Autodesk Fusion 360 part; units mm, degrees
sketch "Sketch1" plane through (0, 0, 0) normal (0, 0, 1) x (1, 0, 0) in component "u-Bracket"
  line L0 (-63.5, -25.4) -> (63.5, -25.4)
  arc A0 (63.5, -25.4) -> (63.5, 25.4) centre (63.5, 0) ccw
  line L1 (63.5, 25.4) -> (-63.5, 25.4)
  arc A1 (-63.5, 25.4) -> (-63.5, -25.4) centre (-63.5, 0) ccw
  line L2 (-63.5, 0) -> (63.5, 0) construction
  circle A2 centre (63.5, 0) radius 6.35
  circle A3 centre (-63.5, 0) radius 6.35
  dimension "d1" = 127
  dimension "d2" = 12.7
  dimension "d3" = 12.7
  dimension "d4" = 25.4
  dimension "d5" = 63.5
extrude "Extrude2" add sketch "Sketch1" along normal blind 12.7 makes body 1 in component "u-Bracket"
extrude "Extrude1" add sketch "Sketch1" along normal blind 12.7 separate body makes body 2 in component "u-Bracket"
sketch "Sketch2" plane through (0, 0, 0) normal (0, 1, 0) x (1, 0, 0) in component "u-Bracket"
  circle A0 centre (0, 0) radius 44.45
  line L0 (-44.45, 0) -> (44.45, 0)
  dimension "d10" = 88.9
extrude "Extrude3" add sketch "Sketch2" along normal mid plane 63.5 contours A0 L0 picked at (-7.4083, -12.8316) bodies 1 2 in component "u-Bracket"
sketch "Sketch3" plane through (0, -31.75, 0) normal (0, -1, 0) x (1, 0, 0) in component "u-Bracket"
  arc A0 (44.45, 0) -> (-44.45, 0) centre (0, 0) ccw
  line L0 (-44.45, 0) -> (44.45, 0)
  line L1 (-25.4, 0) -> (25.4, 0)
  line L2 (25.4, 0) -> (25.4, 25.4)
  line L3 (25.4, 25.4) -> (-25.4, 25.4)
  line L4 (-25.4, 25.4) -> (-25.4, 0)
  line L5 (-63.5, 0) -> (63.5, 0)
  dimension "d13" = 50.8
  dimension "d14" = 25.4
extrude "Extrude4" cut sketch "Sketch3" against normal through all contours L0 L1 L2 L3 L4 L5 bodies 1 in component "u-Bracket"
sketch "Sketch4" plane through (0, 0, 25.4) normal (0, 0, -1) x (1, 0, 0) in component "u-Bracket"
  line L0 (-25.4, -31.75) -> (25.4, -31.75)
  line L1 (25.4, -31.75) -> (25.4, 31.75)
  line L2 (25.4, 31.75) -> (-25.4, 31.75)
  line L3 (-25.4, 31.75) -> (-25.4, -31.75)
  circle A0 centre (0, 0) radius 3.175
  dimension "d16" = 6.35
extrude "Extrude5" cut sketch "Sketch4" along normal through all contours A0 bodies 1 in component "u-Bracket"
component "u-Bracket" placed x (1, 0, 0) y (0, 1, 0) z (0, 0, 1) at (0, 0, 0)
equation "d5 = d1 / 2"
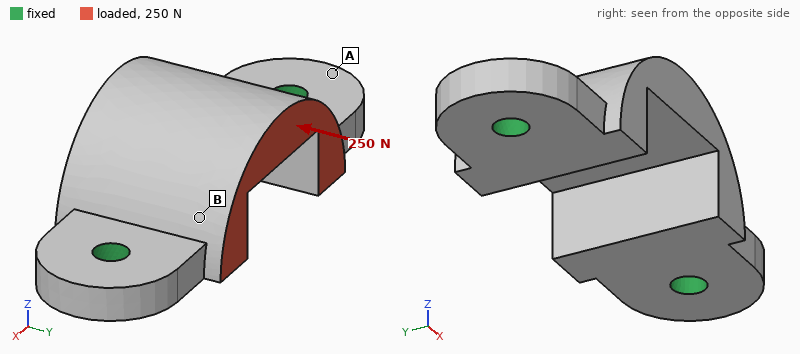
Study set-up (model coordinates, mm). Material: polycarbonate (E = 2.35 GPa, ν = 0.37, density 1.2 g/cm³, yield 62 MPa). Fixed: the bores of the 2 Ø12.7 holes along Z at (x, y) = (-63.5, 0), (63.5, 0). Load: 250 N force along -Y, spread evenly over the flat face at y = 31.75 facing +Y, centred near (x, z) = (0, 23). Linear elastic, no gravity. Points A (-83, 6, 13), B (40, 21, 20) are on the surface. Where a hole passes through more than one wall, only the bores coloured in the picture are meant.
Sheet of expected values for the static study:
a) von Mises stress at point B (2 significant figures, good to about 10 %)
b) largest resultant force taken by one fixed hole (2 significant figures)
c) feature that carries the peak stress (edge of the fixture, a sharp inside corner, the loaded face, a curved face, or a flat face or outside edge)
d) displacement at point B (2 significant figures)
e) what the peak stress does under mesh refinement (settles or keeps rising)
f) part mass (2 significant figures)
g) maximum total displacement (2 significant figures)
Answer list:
0.56 MPa
130 N
edge of the fixture
0.052 mm
keeps rising
200 g
0.11 mm
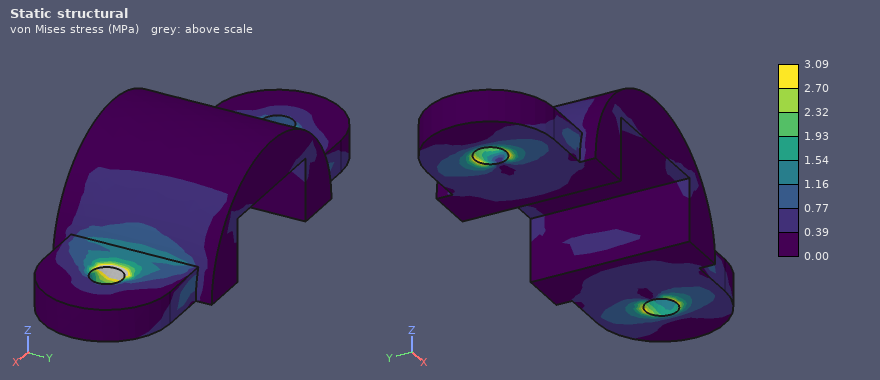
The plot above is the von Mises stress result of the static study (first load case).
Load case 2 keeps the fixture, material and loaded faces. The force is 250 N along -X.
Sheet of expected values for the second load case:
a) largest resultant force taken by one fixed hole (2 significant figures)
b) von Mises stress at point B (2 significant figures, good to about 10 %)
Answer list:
140 N
0.38 MPa
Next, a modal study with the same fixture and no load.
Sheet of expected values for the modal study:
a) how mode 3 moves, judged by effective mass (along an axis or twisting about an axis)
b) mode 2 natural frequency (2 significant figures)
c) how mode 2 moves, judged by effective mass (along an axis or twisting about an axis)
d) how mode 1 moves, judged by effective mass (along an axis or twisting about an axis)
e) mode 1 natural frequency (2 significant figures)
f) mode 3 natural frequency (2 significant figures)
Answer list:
along X
1500 Hz
along Z
along Y
720 Hz
1600 Hz
